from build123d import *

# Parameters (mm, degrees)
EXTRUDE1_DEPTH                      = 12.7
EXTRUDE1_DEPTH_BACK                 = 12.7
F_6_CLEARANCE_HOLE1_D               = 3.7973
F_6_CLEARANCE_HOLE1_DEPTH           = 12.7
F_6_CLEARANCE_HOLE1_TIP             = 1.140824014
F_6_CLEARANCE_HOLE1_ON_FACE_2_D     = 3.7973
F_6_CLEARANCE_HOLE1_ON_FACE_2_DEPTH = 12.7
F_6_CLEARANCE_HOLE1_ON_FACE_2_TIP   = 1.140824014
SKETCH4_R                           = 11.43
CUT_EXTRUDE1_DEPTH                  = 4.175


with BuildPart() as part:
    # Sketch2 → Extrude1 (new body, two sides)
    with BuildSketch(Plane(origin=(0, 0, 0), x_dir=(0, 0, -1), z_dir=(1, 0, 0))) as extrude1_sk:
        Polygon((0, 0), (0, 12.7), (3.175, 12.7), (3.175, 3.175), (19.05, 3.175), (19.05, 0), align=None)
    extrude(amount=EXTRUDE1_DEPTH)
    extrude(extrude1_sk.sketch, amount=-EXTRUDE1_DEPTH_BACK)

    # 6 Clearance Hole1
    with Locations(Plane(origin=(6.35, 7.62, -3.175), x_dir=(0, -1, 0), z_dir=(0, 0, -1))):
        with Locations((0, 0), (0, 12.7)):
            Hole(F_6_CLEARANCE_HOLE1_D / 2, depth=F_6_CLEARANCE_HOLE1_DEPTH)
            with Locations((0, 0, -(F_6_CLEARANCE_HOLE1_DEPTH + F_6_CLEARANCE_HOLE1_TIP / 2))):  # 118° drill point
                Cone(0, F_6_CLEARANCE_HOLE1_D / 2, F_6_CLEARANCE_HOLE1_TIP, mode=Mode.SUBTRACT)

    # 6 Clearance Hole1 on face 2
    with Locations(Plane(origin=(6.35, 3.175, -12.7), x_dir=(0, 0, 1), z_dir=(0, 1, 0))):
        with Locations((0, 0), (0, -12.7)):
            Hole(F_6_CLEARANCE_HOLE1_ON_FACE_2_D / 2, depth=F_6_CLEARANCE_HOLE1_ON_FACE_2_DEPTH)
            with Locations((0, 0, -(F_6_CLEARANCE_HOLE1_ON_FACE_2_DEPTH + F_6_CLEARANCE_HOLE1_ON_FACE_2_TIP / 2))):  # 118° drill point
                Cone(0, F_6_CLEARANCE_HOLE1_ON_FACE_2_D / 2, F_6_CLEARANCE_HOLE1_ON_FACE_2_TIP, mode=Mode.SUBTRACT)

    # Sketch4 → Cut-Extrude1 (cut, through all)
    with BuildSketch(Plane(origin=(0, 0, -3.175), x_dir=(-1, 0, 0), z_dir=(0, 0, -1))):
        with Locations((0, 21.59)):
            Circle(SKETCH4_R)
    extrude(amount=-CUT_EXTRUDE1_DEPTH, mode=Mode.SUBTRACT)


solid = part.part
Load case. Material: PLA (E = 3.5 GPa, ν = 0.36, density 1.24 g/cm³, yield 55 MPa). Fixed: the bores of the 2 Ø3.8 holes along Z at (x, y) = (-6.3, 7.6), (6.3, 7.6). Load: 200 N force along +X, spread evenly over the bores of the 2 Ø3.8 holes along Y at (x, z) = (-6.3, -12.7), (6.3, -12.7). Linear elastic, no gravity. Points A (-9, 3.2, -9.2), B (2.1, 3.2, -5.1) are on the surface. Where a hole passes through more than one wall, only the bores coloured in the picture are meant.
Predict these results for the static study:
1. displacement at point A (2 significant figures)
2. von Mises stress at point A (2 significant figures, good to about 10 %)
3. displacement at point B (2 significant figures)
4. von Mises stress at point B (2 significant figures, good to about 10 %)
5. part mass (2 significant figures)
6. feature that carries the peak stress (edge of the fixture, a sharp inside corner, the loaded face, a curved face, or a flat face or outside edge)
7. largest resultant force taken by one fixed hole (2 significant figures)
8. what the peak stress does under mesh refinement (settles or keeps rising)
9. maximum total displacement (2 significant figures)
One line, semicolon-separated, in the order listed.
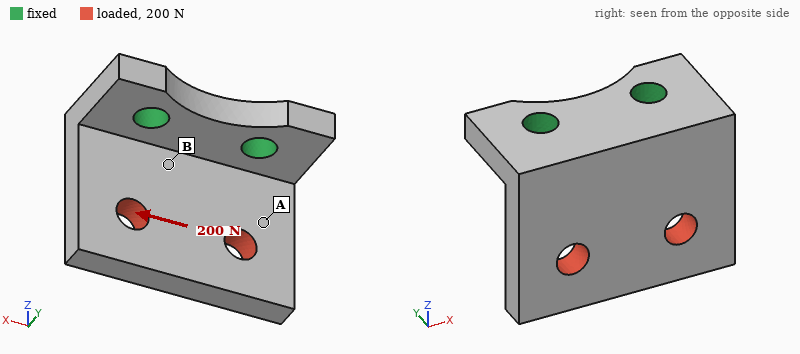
0.12 mm; 6.6 MPa; 0.047 mm; 13 MPa; 2.6 g; edge of the fixture; 180 N; keeps rising; 0.23 mm
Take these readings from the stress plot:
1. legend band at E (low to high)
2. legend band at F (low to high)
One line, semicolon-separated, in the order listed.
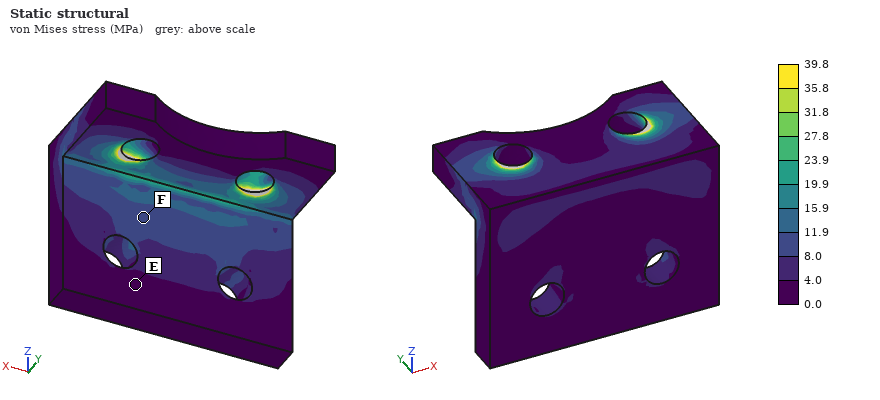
0.0 to 4.0 MPa; 8.0 to 11.9 MPa
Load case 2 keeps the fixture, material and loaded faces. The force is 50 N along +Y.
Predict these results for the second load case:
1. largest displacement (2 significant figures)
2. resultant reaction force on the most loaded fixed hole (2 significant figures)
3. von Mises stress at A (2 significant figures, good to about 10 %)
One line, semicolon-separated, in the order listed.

0.35 mm; 26 N; 4.3 MPa
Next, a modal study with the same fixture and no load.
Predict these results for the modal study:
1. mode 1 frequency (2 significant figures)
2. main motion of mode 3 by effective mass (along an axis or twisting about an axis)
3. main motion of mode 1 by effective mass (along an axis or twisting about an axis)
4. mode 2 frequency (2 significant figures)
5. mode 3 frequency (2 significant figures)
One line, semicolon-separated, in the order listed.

2100 Hz; along X; along Y; 3900 Hz; 5600 Hz
